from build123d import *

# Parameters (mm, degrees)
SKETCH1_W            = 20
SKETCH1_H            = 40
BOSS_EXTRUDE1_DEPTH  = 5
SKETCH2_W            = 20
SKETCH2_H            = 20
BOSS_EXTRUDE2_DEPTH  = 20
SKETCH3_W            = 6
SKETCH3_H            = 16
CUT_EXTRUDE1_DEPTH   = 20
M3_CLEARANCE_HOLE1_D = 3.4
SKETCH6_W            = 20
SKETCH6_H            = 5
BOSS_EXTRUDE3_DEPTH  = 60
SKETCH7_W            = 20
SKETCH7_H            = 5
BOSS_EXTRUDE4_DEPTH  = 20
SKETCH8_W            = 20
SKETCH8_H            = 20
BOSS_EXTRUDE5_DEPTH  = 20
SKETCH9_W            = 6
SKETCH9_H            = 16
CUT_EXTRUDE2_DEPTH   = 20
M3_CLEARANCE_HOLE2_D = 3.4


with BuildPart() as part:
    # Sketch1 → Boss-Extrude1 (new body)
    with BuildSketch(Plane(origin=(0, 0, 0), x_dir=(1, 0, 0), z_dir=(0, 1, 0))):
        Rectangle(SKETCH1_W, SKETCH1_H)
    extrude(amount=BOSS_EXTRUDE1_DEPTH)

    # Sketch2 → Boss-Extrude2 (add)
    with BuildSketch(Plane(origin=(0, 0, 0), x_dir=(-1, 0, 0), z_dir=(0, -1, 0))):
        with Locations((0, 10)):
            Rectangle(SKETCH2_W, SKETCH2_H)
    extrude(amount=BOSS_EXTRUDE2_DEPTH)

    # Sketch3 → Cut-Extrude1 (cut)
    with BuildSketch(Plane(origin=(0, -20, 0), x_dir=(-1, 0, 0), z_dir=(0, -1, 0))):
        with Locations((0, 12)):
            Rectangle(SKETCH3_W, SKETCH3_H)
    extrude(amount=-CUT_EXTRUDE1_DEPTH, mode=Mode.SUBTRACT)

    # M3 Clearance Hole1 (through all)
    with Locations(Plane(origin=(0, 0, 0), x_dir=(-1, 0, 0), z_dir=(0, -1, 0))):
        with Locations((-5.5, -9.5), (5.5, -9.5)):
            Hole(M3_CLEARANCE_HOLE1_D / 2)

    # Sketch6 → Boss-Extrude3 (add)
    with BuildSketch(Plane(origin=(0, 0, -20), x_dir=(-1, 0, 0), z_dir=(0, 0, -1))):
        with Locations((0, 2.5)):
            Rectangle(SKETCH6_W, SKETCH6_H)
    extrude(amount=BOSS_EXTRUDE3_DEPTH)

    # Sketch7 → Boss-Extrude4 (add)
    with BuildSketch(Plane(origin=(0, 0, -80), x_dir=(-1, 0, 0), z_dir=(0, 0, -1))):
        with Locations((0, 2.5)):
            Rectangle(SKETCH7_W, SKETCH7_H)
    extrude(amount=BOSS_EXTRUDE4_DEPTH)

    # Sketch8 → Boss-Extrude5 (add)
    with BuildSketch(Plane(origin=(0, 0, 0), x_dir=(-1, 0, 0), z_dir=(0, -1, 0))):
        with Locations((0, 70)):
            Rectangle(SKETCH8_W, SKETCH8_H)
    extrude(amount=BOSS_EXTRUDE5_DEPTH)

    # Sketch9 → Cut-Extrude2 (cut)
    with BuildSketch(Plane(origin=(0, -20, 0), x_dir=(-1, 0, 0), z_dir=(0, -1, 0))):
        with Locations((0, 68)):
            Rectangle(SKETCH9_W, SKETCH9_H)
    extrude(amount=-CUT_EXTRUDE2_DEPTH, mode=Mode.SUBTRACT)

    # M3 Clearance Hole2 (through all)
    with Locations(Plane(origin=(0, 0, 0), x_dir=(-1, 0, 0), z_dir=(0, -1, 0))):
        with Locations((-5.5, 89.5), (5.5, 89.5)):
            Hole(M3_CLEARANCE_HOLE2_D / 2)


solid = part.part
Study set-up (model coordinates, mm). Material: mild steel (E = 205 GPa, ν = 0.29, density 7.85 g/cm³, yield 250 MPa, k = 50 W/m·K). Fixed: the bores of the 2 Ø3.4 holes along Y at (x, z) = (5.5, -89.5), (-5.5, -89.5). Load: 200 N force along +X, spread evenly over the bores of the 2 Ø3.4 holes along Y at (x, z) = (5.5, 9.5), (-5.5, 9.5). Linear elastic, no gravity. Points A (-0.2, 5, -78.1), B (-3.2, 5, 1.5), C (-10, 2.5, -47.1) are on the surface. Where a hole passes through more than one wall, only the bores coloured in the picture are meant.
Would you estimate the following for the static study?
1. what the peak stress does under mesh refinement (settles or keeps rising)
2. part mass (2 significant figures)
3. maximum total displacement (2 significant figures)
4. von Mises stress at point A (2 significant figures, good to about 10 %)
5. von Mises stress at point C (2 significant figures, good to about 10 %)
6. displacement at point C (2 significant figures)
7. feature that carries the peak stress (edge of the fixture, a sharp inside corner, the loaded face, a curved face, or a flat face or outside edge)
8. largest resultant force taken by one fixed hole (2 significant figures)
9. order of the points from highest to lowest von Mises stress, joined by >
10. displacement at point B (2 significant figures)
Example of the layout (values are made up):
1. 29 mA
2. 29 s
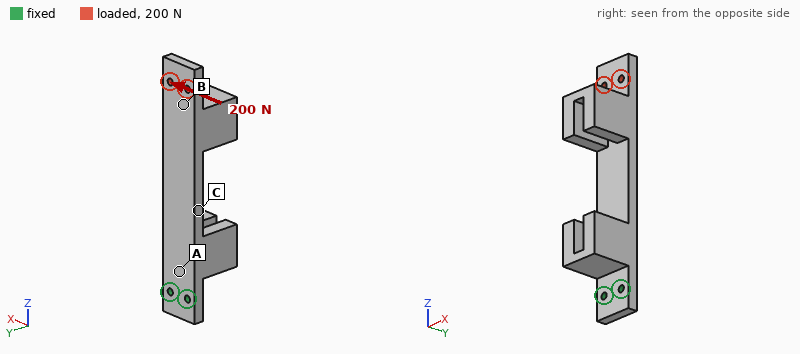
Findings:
1. keeps rising
2. 190 g
3. 0.10 mm
4. 17 MPa
5. 34 MPa
6. 0.023 mm
7. edge of the fixture
8. 1.6 kN
9. C > A > B
10. 0.078 mm
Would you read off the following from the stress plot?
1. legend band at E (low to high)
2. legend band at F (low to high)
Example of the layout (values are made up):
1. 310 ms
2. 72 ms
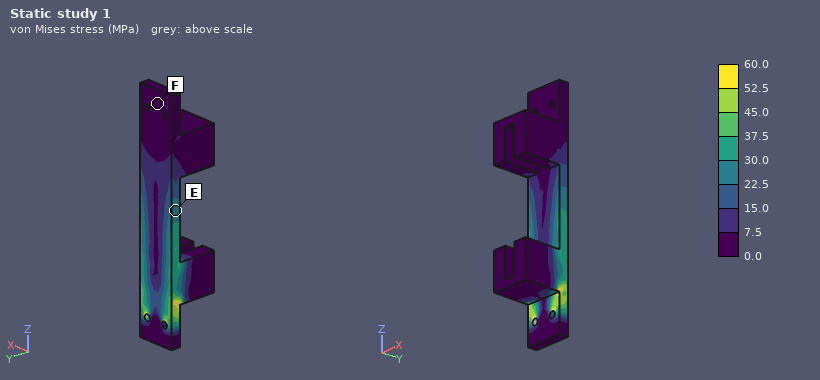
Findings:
1. 22.5 to 30.0 MPa
2. 0.0 to 7.5 MPa
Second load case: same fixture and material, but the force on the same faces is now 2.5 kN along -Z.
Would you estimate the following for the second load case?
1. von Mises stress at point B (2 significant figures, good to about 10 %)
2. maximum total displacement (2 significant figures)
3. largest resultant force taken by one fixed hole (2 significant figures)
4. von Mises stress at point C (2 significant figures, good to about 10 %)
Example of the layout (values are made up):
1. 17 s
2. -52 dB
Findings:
1. 26 MPa
2. 35 µm
3. 1.3 kN
4. 25 MPa
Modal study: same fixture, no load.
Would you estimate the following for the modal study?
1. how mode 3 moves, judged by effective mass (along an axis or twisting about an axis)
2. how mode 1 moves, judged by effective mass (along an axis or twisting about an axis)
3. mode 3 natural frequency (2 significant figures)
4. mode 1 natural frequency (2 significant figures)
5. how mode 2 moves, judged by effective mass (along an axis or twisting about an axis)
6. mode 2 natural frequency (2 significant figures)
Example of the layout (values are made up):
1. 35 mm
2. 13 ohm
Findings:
1. along Y
2. along Y
3. 1700 Hz
4. 300 Hz
5. along X
6. 950 Hz
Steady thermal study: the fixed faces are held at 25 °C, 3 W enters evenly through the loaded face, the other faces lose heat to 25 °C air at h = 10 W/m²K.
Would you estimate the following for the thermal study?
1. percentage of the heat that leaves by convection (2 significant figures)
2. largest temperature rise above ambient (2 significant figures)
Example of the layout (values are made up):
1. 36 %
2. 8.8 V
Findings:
1. 50 %
2. 33 K
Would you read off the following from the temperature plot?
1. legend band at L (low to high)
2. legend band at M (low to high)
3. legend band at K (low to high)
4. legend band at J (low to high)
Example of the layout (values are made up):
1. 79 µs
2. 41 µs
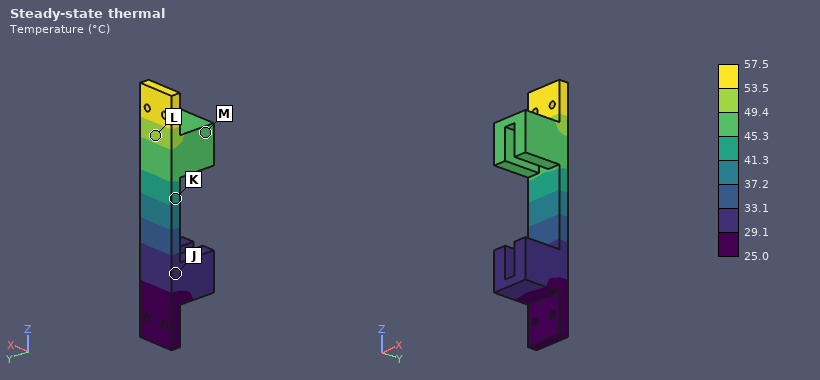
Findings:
1. 49.4 to 53.5 °C
2. 45.3 to 49.4 °C
3. 41.3 to 45.3 °C
4. 29.1 to 33.1 °C
